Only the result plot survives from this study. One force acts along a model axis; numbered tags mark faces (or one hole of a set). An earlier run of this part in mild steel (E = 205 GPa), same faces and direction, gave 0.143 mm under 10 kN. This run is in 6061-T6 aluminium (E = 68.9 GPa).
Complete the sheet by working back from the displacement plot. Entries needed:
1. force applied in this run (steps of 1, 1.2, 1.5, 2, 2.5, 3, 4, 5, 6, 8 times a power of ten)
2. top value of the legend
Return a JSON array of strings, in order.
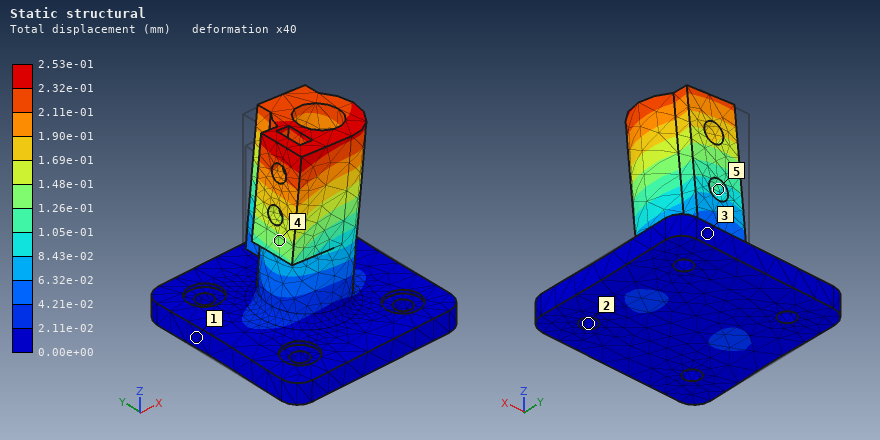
["6 kN", "2.53e-01 mm"]
